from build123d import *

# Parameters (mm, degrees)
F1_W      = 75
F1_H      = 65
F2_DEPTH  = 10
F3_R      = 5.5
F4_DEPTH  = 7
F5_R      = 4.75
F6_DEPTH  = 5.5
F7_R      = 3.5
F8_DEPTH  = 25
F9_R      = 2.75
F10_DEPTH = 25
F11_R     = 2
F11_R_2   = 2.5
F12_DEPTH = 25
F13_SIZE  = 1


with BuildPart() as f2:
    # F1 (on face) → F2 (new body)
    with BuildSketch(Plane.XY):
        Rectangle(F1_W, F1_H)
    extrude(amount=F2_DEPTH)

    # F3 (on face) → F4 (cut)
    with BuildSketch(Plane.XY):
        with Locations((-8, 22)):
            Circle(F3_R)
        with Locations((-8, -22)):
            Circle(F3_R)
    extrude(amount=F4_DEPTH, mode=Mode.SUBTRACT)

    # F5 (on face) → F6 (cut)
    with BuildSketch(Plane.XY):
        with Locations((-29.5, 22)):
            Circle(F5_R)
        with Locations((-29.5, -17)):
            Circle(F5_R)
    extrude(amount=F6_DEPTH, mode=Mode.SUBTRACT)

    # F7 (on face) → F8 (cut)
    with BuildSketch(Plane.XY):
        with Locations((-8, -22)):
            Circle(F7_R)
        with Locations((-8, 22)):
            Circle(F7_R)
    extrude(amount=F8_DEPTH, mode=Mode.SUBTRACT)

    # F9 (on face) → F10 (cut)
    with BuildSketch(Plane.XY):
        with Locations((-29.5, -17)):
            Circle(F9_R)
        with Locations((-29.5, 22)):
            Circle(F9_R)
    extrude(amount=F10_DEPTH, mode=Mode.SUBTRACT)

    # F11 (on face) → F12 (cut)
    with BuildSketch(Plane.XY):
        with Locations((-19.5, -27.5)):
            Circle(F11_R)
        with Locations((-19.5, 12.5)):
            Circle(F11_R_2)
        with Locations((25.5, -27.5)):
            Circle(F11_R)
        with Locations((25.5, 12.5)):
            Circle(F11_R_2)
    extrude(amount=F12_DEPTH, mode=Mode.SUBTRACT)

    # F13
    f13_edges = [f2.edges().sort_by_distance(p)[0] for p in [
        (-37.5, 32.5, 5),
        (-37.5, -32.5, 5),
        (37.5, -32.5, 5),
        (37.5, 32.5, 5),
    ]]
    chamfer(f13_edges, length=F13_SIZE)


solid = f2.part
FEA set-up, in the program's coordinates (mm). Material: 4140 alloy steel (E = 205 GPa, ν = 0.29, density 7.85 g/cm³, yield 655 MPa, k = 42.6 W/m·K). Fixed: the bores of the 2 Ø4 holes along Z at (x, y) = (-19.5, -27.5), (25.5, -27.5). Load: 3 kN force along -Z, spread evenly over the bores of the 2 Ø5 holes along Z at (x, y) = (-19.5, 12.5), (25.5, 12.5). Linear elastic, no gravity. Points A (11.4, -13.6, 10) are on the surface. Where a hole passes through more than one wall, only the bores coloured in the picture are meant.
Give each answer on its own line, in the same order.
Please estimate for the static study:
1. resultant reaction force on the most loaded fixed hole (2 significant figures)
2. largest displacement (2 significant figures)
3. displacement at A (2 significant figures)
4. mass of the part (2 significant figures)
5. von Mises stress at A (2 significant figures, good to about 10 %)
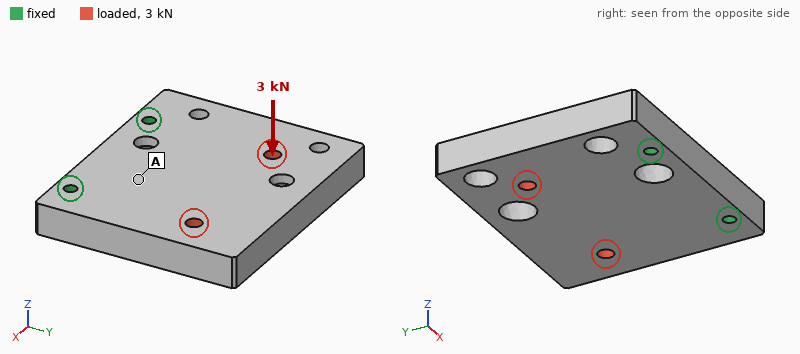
1.6 kN
0.15 mm
0.025 mm
360 g
54 MPa
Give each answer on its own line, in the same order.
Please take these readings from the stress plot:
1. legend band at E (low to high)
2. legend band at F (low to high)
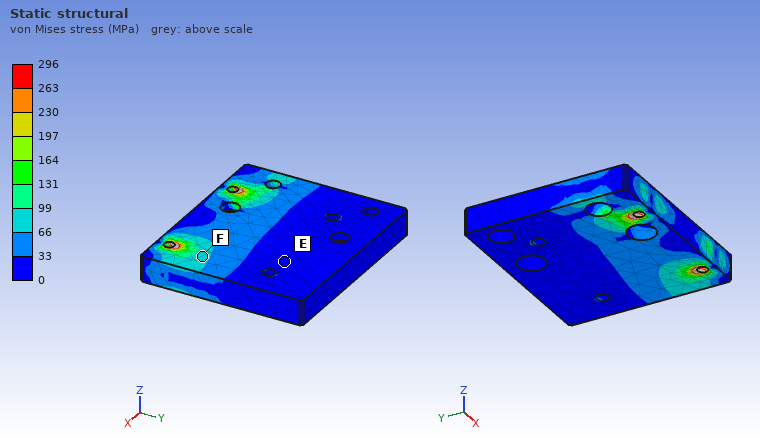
0 to 33 MPa
66 to 99 MPa
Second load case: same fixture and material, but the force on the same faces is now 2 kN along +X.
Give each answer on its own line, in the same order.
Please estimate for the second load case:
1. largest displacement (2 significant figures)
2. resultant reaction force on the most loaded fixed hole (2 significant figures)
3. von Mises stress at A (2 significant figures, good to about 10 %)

5.5 µm
2.0 kN
8.3 MPa
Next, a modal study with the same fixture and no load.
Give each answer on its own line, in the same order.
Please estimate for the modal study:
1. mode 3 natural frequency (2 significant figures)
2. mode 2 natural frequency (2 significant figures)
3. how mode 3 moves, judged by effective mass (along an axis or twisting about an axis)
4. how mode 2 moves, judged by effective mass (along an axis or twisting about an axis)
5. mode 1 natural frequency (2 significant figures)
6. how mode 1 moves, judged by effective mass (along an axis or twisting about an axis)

7100 Hz
4000 Hz
along X
twisting about Y
1800 Hz
along Z
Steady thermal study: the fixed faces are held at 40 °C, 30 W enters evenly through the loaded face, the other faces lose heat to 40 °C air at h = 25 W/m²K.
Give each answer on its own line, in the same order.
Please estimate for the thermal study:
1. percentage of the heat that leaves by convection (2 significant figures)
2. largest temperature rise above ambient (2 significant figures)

27 %
45 K
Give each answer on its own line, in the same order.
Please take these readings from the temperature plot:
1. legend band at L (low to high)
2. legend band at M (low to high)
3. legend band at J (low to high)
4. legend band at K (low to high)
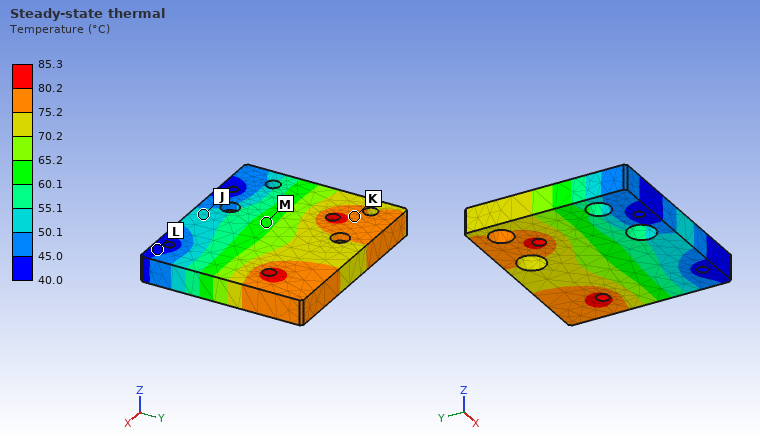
40.0 to 45.0 °C
60.1 to 65.2 °C
50.1 to 55.1 °C
75.2 to 80.2 °C
